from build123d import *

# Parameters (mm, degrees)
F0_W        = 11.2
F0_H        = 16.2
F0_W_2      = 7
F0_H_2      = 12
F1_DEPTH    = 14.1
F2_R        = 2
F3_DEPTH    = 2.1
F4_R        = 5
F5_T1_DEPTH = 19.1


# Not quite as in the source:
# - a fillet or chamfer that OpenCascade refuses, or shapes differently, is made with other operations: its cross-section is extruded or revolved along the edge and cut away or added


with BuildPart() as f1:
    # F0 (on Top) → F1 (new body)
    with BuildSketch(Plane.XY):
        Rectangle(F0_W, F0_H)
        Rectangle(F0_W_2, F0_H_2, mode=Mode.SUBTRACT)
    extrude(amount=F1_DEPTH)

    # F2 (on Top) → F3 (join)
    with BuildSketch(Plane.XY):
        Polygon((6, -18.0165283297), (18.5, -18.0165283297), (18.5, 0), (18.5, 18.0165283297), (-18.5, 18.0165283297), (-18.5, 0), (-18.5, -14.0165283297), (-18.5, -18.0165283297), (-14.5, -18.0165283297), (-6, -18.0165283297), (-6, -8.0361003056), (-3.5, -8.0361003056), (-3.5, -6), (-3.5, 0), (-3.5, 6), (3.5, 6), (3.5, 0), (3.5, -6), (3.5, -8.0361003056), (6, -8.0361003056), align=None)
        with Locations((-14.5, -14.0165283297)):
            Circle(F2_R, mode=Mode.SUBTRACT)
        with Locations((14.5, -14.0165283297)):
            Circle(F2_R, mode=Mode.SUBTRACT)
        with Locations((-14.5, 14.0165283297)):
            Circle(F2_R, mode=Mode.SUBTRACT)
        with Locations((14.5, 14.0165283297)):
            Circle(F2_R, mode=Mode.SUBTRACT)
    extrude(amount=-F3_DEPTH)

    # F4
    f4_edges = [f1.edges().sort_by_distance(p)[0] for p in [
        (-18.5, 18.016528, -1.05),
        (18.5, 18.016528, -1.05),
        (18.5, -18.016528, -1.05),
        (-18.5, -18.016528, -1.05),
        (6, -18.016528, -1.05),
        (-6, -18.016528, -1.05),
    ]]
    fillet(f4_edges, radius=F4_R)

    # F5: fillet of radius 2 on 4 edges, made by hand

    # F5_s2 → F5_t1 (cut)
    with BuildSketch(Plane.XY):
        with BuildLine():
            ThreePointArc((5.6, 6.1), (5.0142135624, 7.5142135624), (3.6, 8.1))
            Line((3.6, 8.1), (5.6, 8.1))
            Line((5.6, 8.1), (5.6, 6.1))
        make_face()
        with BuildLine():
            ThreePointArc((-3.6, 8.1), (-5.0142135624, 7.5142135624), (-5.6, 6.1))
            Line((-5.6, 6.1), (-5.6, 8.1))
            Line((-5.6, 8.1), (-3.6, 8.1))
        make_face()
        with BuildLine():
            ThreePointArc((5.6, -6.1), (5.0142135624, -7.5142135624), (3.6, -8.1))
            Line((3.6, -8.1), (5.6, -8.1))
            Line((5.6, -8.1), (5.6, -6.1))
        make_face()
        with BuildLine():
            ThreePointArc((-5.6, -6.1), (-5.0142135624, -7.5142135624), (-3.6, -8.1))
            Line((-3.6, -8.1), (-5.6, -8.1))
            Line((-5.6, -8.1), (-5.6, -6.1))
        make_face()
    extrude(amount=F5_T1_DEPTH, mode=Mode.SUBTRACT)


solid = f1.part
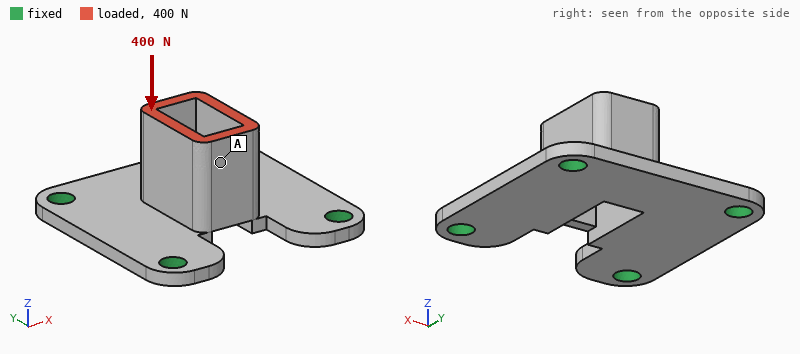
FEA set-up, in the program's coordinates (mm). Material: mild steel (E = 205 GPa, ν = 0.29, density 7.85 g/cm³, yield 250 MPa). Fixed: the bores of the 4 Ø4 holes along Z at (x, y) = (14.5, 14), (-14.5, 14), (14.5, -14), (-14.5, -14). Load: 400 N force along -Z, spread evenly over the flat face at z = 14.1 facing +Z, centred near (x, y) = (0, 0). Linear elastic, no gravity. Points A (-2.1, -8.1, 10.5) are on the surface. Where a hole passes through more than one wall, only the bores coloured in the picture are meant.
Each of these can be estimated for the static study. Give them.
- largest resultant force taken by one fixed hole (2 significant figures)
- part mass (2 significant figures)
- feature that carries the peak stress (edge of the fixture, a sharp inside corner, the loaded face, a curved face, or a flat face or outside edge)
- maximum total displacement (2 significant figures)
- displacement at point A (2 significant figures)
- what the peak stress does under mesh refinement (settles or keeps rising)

140 N
27 g
edge of the fixture
13 µm
13 µm
keeps rising
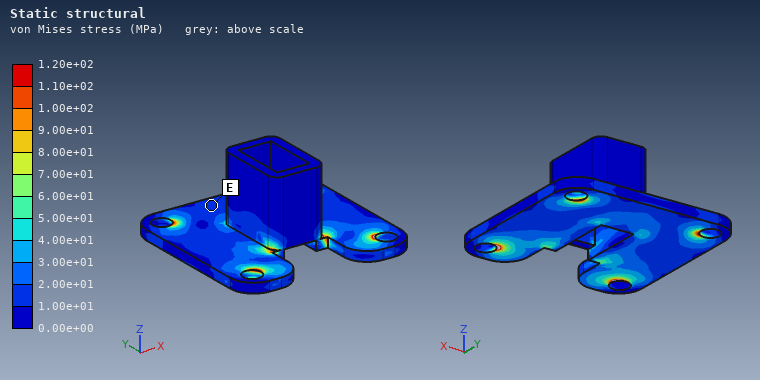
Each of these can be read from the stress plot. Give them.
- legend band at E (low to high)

1.00e+01 to 2.00e+01 MPa
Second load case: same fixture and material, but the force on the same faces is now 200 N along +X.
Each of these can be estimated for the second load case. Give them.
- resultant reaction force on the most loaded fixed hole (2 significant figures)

110 N
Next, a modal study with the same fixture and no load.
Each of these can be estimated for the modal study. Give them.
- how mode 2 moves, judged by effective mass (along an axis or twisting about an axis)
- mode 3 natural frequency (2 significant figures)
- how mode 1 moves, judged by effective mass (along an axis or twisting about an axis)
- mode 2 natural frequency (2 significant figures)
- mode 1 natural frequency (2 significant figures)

along X
9200 Hz
along Z
8700 Hz
7700 Hz
